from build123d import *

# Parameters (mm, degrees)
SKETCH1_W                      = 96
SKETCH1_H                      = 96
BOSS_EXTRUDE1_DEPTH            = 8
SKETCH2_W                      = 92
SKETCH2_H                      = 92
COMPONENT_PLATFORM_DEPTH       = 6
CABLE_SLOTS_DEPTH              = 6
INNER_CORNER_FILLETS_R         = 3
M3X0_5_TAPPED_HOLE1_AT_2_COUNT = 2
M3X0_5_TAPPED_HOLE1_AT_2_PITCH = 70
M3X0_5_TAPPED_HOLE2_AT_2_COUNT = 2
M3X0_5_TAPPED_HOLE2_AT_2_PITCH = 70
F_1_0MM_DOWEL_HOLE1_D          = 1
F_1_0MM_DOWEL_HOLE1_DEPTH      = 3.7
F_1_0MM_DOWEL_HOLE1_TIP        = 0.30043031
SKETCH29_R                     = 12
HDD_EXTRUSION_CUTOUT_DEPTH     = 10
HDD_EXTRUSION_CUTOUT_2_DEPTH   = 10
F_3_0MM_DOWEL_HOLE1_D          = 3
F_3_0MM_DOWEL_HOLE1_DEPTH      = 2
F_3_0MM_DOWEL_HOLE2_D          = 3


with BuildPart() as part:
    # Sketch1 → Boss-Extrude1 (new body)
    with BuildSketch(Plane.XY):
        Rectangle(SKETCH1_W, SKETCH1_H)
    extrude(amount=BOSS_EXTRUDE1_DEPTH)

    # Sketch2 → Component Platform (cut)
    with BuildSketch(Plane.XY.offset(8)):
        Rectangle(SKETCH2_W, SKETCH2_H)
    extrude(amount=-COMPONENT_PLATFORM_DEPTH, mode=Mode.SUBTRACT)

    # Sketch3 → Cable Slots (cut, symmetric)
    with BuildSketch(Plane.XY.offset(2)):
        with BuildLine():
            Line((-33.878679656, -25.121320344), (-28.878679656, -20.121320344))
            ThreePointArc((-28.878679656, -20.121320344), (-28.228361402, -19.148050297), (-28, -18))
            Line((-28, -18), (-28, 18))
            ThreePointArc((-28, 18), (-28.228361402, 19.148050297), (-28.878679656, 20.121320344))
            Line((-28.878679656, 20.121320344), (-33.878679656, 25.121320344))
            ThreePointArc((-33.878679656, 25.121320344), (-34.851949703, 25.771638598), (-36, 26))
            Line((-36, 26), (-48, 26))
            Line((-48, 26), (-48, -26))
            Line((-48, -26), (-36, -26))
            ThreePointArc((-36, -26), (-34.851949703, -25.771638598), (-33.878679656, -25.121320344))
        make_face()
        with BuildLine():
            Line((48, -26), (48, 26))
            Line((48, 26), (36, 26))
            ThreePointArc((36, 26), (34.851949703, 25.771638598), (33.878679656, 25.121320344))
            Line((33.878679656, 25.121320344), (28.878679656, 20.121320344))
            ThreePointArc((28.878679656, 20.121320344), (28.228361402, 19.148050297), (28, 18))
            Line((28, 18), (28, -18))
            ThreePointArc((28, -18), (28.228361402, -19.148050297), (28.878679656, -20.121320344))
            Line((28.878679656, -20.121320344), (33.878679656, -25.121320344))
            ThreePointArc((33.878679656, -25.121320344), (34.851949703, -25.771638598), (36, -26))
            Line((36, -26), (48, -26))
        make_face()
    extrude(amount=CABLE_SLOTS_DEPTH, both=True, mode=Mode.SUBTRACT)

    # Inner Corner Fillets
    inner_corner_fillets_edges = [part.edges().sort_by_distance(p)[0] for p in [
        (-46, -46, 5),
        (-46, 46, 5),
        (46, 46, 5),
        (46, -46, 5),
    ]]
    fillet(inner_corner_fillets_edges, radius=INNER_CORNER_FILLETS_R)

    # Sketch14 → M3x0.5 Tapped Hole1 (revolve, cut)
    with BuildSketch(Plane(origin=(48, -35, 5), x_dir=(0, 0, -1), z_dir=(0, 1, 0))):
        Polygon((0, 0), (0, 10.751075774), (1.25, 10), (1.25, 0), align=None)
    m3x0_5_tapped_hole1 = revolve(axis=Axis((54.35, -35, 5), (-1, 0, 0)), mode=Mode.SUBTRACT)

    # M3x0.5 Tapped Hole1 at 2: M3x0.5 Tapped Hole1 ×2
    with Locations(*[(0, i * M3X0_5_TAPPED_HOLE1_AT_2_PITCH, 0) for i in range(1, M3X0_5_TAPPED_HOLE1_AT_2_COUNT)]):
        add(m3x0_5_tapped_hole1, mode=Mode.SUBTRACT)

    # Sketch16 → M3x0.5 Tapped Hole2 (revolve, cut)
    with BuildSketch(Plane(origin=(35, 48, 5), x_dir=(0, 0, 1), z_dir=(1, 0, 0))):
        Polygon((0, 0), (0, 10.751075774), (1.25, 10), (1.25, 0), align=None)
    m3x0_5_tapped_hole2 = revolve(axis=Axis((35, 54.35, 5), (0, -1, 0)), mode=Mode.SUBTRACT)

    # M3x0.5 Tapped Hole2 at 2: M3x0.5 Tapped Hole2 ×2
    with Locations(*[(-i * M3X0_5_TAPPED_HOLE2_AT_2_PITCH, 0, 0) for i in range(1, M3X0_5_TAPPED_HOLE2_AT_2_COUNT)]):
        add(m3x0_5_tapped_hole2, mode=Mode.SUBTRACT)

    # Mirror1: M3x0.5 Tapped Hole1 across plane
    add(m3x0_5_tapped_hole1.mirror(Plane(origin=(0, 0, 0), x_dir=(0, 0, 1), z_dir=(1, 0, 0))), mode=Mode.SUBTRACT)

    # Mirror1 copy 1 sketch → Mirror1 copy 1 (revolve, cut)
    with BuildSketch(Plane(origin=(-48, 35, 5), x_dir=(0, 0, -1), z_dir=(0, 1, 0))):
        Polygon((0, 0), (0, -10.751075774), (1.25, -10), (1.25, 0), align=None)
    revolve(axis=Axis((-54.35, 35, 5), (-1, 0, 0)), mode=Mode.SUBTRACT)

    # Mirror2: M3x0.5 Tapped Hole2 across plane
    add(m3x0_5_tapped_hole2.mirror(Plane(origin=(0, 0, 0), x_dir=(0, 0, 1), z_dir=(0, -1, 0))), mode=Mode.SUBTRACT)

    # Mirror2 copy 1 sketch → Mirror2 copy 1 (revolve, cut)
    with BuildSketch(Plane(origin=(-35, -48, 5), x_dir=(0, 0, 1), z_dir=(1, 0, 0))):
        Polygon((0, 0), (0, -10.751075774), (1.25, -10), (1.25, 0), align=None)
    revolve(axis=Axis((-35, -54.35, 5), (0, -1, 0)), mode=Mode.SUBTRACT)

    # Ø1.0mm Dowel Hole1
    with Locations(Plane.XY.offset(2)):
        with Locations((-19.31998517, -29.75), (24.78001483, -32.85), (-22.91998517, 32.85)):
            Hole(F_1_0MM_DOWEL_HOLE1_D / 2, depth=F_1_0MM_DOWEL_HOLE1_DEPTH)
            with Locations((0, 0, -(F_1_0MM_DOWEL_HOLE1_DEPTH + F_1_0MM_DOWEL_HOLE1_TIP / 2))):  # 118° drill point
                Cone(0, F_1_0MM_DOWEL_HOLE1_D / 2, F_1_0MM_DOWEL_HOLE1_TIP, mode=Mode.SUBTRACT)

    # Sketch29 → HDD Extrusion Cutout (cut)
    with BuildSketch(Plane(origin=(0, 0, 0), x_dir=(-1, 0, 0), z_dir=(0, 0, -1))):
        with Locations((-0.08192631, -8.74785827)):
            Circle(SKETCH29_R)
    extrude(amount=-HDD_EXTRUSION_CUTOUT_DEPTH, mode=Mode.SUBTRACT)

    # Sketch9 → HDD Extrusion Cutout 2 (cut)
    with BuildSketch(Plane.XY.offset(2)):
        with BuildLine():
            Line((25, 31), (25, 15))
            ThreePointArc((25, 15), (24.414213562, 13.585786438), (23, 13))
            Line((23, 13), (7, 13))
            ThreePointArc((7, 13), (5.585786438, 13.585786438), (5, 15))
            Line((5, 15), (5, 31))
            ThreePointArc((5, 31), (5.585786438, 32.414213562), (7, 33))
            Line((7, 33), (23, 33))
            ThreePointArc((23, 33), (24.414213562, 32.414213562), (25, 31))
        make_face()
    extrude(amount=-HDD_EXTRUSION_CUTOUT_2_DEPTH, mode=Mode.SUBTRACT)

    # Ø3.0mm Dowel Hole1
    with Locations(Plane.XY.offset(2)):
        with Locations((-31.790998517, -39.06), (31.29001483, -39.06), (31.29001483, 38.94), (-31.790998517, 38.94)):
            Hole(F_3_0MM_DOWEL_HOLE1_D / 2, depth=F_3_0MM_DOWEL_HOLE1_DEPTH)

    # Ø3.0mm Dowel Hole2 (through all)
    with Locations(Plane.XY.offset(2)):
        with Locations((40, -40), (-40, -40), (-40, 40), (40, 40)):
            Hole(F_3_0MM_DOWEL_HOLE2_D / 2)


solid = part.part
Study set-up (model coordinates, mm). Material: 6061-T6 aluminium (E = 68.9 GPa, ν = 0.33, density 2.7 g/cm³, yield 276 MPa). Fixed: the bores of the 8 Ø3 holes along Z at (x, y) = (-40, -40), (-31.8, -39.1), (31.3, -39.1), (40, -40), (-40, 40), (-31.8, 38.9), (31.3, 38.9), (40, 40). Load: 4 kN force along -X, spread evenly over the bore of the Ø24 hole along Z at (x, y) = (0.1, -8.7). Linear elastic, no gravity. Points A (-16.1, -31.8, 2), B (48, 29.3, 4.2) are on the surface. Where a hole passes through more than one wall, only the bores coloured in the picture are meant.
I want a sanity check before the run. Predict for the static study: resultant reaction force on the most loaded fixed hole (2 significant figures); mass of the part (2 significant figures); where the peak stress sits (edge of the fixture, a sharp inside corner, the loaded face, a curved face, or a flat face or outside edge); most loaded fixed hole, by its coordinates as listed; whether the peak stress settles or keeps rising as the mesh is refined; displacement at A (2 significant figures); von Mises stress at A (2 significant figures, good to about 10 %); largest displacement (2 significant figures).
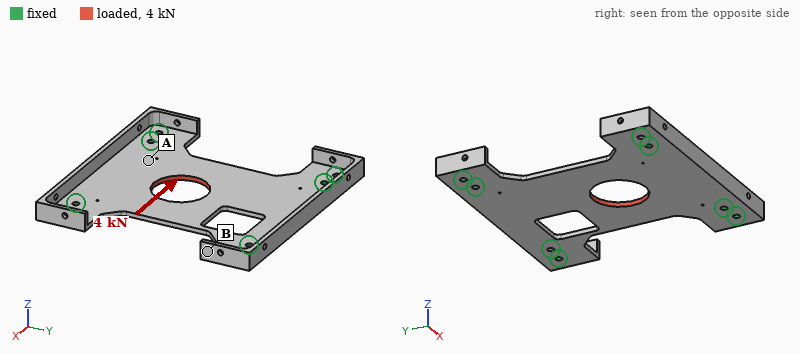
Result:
1.0 kN
43 g
a sharp inside corner
(-31.8, -39.1)
keeps rising
9.5 µm
28 MPa
45 µm
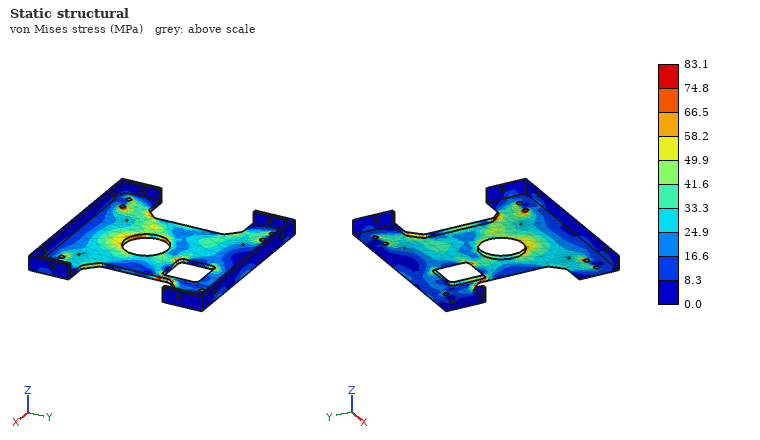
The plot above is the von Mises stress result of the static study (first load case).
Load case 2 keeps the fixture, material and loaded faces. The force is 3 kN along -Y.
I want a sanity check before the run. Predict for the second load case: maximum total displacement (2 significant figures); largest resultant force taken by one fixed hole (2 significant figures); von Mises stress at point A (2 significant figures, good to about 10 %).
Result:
29 µm
1000 N
22 MPa
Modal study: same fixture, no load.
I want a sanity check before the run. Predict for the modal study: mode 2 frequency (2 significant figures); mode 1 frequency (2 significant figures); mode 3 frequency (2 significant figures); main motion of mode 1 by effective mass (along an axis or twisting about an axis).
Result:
2500 Hz
1400 Hz
3200 Hz
along Z
